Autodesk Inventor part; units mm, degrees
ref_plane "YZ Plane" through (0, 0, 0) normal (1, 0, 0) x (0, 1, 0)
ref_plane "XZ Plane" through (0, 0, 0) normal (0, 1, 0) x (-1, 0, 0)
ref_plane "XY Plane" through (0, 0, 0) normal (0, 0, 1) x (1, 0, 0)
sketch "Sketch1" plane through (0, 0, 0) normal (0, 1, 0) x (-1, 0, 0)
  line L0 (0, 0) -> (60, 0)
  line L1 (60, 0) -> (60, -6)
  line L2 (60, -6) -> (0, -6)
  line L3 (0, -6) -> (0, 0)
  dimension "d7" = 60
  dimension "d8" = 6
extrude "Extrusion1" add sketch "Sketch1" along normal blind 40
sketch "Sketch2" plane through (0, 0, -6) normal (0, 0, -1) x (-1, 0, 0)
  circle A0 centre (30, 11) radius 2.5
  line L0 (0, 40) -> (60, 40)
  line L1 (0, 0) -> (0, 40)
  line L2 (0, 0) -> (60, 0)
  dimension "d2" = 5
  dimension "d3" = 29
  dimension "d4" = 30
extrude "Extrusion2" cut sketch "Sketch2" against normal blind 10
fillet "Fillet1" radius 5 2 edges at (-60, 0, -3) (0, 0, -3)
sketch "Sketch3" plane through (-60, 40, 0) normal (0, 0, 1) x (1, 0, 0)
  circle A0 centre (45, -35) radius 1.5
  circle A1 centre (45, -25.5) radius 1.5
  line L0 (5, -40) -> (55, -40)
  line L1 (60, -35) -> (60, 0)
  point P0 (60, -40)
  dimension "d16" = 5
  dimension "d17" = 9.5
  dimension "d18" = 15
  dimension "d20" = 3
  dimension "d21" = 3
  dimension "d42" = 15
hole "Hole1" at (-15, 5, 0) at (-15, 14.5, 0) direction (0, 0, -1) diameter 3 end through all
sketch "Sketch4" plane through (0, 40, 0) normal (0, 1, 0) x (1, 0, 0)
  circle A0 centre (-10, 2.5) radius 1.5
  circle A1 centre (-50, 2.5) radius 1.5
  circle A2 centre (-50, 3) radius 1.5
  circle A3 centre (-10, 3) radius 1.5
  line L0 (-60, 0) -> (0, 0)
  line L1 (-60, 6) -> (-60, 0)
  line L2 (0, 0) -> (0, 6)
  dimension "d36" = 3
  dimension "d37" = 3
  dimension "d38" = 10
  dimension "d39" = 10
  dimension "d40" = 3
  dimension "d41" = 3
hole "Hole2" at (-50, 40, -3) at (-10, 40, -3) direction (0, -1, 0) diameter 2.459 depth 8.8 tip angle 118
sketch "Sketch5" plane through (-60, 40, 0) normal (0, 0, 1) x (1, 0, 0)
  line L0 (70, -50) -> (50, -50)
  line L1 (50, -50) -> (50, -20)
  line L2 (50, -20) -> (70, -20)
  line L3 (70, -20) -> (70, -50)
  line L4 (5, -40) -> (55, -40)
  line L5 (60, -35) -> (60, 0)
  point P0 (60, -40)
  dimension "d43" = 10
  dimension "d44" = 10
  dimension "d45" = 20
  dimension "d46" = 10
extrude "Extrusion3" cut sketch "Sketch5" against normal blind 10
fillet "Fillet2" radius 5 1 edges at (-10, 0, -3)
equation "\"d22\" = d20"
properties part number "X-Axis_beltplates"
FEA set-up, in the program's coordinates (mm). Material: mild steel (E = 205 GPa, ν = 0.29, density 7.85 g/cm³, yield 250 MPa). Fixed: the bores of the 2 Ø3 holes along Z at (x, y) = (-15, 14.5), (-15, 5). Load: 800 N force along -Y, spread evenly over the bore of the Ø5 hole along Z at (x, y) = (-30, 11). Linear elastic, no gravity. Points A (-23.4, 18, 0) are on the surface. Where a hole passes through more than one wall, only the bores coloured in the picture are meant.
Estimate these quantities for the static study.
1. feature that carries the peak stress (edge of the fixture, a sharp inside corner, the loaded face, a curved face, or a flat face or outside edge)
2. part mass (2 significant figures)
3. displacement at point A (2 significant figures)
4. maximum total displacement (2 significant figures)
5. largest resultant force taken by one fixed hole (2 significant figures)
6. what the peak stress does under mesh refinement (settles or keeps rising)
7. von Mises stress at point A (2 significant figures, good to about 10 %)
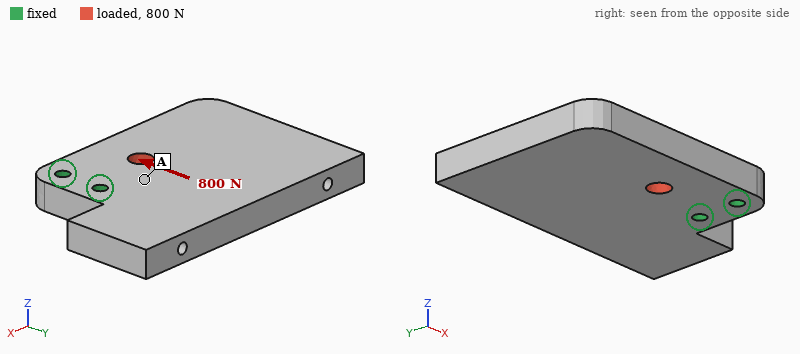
edge of the fixture
100 g
1.8 µm
8.7 µm
1.1 kN
keeps rising
8.6 MPa
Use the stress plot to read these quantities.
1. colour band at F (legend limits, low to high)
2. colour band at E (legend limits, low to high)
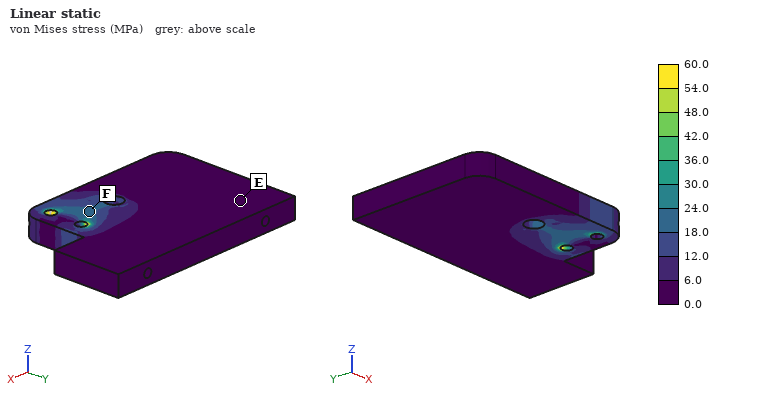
18.0 to 24.0 MPa
0.0 to 6.0 MPa
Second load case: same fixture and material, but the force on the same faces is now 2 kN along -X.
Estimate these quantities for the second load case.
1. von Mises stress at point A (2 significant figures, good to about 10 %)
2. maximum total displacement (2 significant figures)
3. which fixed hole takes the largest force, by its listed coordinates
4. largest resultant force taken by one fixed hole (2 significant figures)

12 MPa
1.9 µm
(-15, 14.5)
1.2 kN
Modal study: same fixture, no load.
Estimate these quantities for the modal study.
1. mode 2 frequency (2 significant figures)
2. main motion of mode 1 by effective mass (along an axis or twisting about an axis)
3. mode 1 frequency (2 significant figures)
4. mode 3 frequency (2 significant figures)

4200 Hz
along Z
1900 Hz
4500 Hz
